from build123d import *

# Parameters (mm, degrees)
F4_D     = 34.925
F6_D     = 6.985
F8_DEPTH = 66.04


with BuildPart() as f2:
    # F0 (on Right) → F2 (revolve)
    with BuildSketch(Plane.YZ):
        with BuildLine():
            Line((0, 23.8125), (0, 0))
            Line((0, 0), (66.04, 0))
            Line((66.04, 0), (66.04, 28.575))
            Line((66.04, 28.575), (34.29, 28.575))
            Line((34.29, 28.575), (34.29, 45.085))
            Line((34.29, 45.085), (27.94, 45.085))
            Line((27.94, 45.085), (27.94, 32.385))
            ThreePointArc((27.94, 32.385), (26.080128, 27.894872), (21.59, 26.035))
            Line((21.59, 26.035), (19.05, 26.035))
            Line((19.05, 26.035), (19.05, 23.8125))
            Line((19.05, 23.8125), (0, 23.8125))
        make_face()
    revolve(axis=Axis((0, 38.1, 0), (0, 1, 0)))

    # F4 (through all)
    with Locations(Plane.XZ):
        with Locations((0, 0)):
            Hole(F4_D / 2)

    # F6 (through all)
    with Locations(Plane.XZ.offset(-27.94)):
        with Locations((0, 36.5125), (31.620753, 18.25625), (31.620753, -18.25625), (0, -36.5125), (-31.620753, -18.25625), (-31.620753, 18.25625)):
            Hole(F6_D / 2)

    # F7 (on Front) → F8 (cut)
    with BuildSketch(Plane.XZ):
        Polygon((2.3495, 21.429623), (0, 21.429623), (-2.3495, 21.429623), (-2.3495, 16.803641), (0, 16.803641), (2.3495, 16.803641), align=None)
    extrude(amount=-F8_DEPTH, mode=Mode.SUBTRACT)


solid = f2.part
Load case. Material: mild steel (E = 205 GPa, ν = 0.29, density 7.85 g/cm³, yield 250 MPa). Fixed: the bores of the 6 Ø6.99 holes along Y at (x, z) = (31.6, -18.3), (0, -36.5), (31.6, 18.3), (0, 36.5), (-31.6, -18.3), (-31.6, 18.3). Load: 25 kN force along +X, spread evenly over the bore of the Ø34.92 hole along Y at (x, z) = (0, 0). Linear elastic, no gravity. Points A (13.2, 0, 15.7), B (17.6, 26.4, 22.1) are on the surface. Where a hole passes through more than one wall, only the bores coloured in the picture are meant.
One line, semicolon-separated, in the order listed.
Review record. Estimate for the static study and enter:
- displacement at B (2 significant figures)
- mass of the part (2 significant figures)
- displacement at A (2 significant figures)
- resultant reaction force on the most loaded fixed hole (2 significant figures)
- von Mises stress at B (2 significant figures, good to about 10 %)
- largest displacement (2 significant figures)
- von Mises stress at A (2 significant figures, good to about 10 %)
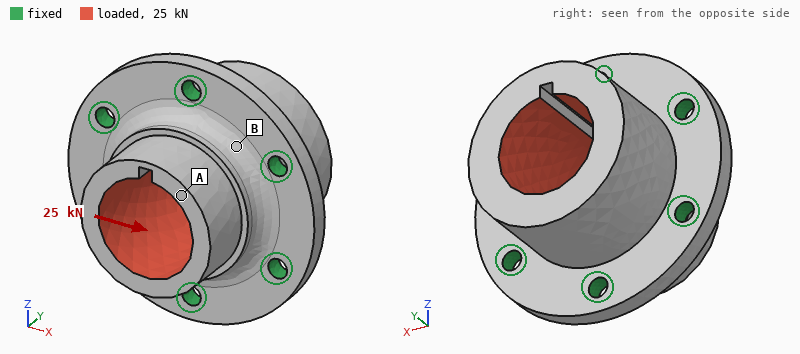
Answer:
1.7 µm; 870 g; 6.2 µm; 5.1 kN; 23 MPa; 7.4 µm; 11 MPa
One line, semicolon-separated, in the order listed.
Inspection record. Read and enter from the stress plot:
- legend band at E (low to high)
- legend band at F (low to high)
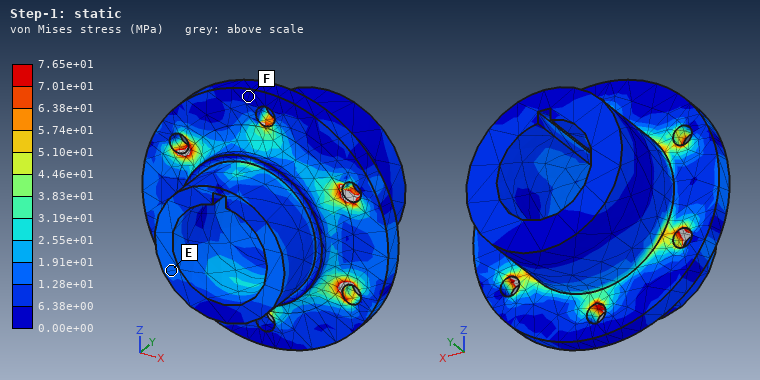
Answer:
1.28e+01 to 1.91e+01 MPa; 0.00e+00 to 6.38e+00 MPa
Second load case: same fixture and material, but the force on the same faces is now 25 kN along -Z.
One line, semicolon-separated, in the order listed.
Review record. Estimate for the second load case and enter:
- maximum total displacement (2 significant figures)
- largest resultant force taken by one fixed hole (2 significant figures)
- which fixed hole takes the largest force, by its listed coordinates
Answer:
7.5 µm; 5.6 kN; (0, -36.5)
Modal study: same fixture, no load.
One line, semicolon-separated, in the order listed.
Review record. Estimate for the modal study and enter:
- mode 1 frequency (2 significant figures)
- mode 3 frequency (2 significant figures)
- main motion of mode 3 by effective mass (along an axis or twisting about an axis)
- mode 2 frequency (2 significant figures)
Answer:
9900 Hz; 11 kHz; along Y; 10000 Hz
